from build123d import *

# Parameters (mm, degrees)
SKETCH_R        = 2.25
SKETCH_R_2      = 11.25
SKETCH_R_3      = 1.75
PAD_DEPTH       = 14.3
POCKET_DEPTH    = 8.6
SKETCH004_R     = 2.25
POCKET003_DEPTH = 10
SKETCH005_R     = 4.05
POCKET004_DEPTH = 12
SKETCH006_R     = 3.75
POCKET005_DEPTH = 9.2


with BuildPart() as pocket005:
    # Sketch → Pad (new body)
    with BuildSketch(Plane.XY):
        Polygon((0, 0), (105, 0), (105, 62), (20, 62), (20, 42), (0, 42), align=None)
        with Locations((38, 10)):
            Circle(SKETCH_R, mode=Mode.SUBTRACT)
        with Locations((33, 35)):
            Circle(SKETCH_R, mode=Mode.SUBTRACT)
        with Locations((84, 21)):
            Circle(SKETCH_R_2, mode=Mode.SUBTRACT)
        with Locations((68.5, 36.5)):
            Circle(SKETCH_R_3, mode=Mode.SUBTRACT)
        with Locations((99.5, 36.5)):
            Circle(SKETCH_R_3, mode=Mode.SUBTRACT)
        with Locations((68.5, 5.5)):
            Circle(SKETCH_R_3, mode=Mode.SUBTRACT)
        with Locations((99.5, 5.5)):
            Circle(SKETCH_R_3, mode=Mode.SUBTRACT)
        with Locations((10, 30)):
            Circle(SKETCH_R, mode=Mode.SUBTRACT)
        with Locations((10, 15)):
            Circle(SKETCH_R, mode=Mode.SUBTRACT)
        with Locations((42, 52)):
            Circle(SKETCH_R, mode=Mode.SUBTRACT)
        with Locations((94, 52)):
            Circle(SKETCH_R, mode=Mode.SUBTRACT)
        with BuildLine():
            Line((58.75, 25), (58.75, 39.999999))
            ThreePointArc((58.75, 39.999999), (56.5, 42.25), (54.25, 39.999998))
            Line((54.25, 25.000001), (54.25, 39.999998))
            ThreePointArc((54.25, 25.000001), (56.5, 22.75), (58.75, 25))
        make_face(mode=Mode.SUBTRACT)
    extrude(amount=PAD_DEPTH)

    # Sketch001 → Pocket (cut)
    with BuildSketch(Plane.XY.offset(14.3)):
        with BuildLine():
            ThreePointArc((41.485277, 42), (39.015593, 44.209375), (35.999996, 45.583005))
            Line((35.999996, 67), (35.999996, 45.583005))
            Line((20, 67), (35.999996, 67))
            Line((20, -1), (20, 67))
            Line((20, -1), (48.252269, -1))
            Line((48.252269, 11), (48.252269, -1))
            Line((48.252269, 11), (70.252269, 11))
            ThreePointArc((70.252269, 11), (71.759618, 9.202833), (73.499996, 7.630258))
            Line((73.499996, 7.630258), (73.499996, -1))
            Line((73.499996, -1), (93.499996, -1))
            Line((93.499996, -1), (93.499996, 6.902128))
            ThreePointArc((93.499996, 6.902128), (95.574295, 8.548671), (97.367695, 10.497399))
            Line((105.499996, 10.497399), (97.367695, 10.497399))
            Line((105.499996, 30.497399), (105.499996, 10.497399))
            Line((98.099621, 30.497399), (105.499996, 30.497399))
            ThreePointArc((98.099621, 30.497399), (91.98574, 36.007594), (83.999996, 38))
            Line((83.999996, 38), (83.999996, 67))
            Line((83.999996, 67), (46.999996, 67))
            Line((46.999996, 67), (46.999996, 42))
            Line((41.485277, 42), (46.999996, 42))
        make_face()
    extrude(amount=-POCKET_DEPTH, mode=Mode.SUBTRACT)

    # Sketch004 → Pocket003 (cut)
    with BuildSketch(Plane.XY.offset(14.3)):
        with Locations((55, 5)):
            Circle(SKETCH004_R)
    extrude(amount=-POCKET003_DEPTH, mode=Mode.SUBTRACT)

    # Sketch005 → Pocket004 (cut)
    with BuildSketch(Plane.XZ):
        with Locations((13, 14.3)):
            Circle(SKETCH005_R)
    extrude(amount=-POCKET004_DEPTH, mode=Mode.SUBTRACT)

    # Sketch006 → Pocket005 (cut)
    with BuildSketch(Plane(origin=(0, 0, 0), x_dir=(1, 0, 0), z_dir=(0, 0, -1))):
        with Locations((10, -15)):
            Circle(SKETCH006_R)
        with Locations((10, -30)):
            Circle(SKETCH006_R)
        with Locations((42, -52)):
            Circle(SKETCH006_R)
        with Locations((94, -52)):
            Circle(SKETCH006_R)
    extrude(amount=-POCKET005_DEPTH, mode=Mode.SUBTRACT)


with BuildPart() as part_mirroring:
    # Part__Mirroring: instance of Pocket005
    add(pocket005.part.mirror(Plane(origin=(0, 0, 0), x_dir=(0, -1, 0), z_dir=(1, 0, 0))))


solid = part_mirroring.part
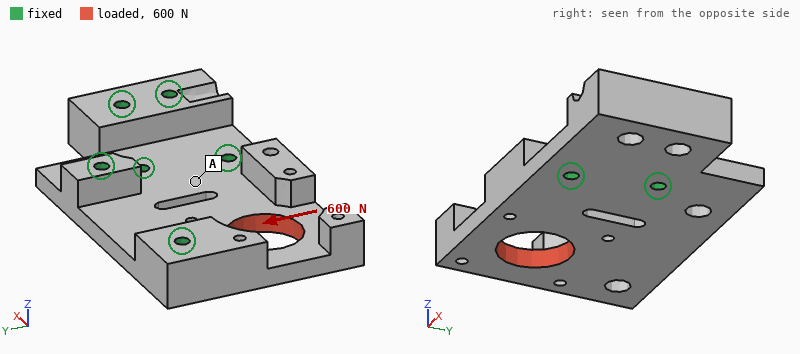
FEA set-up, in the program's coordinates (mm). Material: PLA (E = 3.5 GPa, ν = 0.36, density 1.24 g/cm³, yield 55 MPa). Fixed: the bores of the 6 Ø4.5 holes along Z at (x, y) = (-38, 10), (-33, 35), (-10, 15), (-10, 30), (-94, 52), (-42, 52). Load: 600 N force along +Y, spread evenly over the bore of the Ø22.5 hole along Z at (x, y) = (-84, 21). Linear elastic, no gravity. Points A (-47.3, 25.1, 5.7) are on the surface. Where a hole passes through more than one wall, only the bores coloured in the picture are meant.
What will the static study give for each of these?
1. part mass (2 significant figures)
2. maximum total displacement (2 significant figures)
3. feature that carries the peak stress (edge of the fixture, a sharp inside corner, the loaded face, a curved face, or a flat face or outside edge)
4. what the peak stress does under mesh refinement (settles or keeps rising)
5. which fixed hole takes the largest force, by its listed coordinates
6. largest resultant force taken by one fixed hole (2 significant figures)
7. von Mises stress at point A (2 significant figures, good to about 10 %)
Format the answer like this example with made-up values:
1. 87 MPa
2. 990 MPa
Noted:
1. 58 g
2. 0.27 mm
3. edge of the fixture
4. keeps rising
5. (-94, 52)
6. 330 N
7. 1.9 MPa
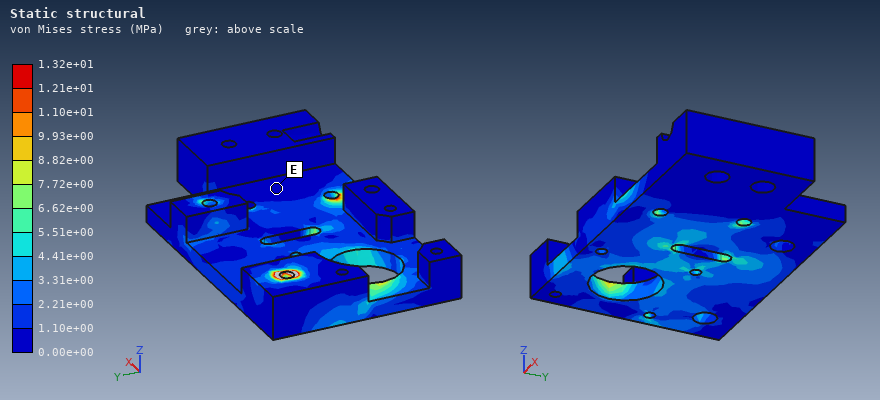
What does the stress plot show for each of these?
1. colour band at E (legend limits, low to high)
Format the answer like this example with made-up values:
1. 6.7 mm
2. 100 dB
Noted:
1. 0.00e+00 to 1.10e+00 MPa
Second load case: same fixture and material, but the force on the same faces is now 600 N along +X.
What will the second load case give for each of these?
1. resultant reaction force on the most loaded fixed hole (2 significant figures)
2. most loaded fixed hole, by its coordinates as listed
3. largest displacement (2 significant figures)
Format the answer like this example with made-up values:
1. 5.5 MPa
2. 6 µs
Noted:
1. 290 N
2. (-38, 10)
3. 69 µm
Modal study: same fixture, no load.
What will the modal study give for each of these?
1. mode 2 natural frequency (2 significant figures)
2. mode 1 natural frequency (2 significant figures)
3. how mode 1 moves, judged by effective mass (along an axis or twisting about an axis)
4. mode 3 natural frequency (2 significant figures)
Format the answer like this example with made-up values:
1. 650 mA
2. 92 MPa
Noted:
1. 2100 Hz
2. 900 Hz
3. along Z
4. 2400 Hz
